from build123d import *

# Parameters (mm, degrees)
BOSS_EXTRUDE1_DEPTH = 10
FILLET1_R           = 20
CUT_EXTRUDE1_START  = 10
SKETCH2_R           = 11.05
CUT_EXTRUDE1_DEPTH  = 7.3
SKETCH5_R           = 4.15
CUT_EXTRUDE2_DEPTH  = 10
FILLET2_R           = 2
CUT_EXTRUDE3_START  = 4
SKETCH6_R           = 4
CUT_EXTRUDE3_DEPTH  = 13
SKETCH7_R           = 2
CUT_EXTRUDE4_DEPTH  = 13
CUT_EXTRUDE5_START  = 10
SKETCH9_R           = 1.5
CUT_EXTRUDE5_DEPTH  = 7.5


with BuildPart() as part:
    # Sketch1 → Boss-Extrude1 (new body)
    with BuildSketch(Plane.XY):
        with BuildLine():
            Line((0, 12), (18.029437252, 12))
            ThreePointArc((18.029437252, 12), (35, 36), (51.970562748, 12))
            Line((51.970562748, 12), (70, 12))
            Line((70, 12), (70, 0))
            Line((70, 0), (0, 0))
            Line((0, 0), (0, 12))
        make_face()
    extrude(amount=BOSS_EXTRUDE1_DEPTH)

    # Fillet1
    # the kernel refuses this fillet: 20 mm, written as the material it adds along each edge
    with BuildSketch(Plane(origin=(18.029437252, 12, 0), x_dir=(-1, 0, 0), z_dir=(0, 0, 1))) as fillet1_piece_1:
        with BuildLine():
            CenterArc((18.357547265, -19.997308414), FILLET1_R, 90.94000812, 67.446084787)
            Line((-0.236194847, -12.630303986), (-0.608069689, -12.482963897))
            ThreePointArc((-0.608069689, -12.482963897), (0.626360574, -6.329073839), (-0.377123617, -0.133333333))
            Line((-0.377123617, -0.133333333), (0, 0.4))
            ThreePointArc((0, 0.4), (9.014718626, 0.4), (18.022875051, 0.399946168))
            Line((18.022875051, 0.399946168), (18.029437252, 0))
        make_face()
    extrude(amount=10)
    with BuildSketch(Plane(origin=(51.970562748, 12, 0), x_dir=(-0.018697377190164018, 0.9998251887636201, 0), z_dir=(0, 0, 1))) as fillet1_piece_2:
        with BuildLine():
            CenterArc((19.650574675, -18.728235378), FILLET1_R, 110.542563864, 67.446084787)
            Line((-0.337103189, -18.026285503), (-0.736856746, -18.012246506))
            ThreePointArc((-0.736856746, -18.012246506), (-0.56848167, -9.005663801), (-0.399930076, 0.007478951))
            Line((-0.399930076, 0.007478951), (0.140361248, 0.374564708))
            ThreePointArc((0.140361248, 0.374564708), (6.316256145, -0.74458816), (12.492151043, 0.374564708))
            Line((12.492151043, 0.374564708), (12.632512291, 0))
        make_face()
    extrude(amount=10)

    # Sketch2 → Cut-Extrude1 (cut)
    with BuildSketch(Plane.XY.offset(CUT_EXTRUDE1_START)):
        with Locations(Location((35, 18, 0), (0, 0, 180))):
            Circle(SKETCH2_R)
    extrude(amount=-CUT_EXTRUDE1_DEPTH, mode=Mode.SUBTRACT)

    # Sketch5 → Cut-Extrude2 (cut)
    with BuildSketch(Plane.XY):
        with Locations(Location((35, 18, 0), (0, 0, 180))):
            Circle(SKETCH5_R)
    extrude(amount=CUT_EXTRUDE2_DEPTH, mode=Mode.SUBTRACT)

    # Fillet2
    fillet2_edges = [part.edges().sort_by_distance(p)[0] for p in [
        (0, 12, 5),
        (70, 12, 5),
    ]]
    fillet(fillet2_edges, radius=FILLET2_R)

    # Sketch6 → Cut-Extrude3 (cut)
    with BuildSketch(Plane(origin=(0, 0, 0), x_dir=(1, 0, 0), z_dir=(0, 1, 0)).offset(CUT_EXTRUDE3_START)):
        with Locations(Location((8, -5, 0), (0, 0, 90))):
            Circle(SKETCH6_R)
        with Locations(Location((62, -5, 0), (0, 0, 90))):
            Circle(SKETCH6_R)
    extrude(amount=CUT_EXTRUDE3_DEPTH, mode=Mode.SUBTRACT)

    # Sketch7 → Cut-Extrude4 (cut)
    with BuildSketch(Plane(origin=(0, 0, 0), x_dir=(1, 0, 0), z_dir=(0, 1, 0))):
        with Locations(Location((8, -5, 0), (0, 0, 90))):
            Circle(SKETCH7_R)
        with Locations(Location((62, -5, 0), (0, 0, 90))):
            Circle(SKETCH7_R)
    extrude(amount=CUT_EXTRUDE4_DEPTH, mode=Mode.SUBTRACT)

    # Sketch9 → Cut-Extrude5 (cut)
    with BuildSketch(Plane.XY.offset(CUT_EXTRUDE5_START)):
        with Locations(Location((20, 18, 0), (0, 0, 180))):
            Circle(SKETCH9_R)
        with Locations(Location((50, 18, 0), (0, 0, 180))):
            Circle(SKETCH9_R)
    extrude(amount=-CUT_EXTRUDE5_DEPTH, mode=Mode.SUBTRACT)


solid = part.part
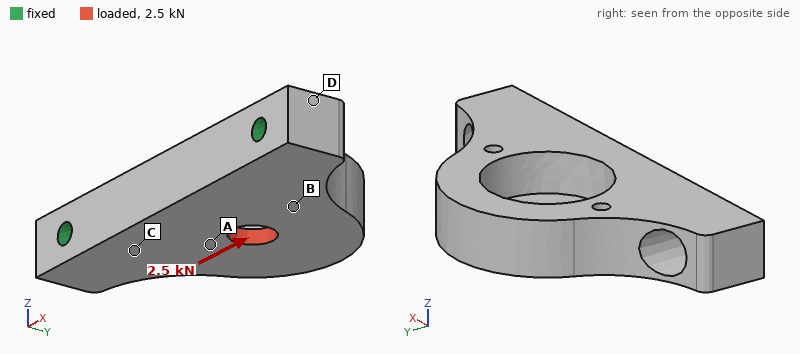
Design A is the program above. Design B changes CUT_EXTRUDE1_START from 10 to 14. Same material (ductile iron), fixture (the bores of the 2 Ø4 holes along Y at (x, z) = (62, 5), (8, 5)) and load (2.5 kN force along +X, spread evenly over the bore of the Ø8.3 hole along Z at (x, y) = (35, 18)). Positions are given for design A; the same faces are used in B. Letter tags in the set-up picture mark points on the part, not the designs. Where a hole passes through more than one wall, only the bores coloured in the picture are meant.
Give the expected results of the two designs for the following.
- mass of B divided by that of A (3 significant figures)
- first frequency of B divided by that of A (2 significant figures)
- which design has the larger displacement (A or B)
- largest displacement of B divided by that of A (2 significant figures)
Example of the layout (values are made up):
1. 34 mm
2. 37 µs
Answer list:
1. 1.11
2. 0.94
3. A
4. 0.66
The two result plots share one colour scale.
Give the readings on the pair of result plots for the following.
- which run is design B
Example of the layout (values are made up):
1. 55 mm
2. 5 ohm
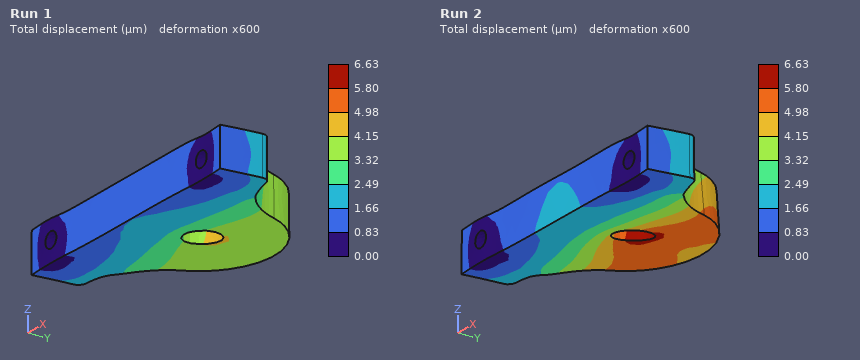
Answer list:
1. Run 1
